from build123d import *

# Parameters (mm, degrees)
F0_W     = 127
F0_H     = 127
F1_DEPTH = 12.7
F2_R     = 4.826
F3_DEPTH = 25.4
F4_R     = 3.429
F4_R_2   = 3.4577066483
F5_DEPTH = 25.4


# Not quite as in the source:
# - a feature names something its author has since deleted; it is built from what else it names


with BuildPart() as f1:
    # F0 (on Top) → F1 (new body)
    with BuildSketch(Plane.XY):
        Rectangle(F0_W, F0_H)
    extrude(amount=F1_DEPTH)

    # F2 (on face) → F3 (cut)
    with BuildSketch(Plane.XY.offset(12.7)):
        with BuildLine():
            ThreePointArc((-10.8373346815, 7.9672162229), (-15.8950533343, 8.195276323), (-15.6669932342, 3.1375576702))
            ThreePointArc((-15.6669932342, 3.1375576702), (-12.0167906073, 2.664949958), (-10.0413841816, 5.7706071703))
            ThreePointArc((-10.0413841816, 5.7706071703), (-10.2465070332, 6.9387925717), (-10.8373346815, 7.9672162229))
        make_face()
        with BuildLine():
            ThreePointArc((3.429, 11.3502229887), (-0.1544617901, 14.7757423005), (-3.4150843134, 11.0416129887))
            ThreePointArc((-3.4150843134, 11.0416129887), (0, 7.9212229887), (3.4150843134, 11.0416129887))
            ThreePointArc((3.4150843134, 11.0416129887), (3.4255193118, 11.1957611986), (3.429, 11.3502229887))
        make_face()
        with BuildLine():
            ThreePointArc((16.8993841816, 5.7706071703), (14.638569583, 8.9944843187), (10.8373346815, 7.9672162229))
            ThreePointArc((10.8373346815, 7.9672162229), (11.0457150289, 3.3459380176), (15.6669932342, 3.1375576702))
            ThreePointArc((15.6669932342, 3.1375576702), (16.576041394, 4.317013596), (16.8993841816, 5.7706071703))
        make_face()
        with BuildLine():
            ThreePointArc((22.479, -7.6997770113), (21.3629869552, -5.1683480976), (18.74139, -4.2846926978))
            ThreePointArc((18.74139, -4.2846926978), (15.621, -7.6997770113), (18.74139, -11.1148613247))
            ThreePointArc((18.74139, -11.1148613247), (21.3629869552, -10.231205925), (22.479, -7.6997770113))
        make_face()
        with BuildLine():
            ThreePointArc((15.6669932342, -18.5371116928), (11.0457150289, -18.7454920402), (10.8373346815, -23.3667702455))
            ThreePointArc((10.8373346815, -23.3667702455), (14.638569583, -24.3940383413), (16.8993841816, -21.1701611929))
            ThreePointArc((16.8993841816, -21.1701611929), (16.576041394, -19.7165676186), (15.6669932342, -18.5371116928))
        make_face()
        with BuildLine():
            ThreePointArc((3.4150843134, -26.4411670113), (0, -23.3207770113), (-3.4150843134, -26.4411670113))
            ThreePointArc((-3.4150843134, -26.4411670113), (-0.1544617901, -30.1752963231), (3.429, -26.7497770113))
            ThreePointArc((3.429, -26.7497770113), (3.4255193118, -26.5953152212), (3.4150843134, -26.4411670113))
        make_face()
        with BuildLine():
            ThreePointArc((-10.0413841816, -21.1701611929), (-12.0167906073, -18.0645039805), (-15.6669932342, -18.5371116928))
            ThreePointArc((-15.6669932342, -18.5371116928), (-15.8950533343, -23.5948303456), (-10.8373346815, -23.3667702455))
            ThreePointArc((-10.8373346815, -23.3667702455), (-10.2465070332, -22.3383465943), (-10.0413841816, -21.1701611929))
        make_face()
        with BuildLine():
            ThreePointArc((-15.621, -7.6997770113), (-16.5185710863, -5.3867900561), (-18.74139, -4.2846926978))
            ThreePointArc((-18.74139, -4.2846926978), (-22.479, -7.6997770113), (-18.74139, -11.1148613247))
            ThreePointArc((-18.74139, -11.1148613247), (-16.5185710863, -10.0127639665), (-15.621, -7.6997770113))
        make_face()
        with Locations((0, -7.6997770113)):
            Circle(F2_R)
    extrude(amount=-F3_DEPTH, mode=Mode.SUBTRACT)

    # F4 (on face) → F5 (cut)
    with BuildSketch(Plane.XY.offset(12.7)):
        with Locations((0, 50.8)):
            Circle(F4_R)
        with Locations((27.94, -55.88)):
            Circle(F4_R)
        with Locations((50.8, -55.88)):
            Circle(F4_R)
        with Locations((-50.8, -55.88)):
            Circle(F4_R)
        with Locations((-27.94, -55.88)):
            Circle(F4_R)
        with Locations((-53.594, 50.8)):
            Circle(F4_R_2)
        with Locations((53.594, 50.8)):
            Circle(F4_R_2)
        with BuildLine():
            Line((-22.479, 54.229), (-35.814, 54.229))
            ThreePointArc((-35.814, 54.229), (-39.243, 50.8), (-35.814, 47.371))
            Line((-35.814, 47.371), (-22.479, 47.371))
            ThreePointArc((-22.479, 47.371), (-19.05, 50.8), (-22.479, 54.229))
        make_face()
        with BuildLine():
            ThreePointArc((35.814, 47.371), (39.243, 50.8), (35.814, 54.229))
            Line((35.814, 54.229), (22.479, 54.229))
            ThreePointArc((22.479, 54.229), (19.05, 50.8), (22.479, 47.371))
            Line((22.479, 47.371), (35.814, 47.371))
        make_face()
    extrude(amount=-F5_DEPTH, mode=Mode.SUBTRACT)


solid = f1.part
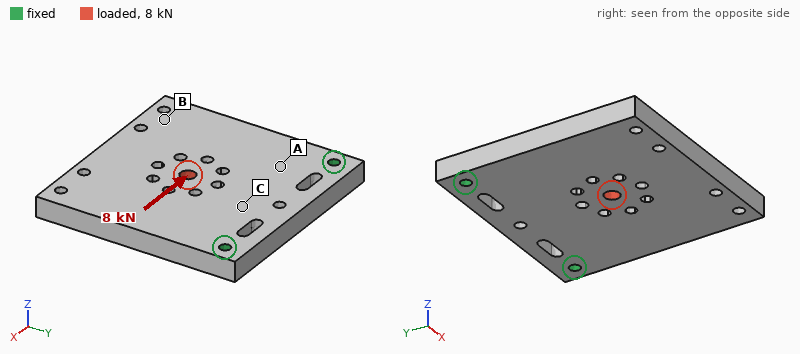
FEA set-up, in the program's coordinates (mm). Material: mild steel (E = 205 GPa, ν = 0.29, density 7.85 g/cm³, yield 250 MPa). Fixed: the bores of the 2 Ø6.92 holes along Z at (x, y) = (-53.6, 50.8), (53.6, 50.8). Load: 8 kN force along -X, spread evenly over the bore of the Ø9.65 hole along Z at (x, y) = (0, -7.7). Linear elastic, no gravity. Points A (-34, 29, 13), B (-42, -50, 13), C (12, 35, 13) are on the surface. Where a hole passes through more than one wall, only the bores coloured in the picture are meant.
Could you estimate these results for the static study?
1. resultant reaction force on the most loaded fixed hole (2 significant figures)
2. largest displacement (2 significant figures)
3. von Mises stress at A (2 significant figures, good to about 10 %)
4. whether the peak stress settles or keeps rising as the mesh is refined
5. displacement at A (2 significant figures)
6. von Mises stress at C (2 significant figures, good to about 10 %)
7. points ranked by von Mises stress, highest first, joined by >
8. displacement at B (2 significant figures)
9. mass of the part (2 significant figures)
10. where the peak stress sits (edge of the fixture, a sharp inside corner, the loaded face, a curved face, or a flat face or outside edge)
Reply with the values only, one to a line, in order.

5.8 kN
9.4 µm
13 MPa
keeps rising
2.9 µm
6.8 MPa
A > C > B
8.7 µm
1.5 kg
edge of the fixture
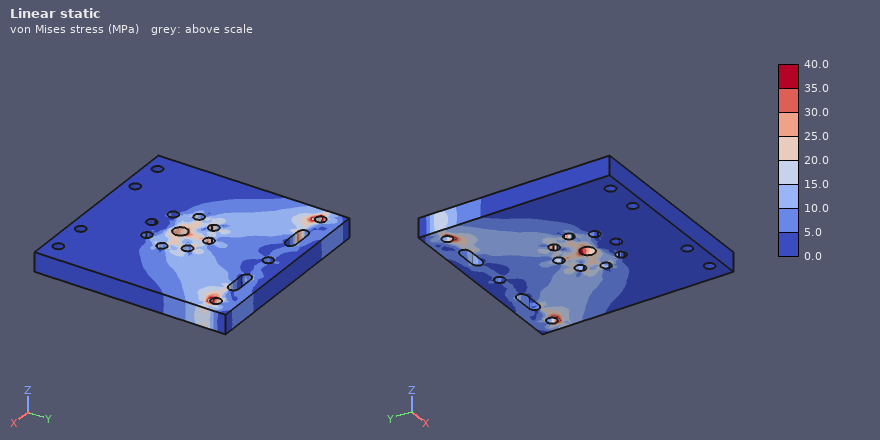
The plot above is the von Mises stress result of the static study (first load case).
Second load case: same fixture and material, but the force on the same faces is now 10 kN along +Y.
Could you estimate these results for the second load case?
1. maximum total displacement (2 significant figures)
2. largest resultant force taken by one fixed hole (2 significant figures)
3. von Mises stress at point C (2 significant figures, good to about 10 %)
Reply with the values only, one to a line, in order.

6.7 µm
5.3 kN
4.1 MPa
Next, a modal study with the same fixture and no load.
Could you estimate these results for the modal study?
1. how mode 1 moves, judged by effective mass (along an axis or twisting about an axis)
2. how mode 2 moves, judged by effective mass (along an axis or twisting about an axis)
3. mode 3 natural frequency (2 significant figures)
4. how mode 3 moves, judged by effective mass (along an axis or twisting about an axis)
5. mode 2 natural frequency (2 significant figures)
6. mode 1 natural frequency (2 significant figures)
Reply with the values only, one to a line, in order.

along Z
twisting about Y
3800 Hz
along Z
1700 Hz
620 Hz
